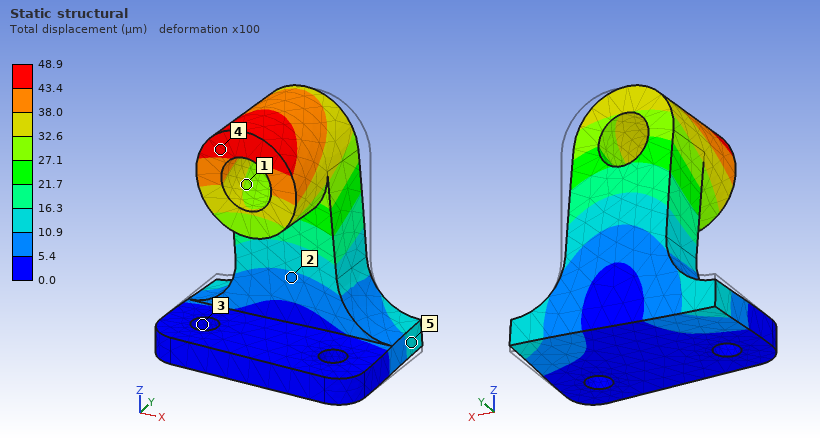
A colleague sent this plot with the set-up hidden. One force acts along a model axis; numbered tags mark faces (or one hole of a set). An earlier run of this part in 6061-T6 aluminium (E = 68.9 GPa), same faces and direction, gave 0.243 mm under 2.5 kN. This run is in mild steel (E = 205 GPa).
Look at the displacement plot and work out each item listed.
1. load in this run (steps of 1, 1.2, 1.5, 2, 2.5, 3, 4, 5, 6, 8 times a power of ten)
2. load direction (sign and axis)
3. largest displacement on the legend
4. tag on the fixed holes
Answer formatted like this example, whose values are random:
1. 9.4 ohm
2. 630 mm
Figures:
1. 1.5 kN
2. -X
3. 48.9 µm
4. 3
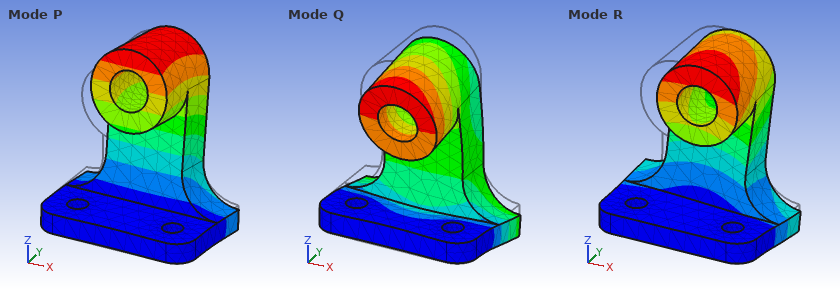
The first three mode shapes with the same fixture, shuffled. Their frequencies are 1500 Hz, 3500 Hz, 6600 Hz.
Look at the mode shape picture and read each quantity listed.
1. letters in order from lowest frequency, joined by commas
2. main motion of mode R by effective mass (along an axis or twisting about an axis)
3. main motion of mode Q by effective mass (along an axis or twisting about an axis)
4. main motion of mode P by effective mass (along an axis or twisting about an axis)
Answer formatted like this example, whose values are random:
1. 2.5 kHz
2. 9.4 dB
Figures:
1. P, R, Q
2. along X
3. along Z
4. along Y
